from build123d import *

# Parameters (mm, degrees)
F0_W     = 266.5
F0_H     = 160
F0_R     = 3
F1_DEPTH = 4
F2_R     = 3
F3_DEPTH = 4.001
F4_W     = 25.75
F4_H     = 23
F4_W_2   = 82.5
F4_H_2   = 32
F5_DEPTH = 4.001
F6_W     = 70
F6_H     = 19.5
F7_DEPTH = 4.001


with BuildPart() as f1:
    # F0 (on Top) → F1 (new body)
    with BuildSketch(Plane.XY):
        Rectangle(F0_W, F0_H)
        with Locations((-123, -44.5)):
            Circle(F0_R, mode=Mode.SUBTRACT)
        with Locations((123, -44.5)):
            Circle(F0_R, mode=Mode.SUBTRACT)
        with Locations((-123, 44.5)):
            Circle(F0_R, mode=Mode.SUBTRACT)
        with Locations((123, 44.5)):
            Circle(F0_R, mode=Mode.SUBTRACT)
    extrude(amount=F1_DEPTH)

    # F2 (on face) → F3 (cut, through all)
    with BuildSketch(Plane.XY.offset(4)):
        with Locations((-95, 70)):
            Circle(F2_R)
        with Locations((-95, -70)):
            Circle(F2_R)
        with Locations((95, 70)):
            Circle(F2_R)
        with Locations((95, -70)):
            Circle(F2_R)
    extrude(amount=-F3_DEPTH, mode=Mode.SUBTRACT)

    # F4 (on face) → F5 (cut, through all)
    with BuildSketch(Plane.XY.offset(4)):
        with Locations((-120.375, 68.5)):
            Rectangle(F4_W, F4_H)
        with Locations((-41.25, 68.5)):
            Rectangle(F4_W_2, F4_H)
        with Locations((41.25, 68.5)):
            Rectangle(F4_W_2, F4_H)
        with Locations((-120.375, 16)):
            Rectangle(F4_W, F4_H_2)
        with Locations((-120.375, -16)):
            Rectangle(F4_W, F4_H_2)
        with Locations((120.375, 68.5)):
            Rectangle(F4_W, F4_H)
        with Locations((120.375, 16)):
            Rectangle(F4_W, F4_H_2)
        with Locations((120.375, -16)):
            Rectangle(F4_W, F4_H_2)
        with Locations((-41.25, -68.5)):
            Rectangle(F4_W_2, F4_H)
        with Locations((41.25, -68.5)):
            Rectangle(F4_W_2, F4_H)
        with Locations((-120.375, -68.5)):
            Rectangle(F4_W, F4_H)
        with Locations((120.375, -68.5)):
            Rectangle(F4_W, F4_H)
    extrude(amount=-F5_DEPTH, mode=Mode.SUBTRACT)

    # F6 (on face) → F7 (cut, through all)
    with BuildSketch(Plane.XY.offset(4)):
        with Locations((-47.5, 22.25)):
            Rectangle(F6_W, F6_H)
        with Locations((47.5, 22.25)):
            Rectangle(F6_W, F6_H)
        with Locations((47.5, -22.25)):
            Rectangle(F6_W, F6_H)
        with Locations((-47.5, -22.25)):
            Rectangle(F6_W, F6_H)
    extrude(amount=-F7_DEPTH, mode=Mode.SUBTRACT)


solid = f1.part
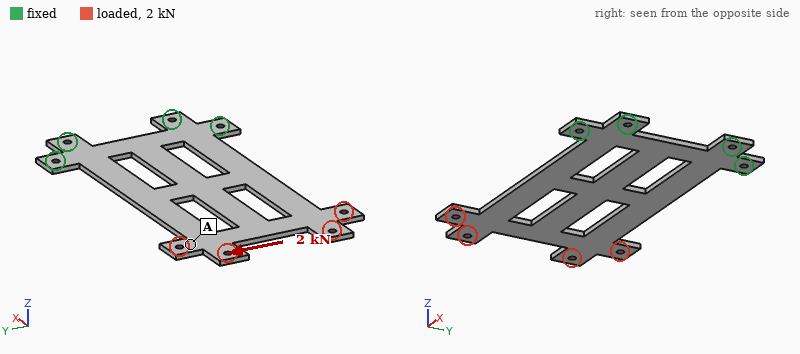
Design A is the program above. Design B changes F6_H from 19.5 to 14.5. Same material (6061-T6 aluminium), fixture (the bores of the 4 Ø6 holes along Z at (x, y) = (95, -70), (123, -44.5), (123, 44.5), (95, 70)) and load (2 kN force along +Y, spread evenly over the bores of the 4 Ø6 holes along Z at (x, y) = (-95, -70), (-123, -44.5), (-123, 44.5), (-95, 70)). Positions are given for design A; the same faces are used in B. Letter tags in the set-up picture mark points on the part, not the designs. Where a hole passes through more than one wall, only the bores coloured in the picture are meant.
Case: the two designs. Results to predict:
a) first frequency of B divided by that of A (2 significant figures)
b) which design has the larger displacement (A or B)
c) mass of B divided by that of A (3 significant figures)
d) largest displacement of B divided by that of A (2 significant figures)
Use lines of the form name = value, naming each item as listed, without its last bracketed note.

first frequency of B divided by that of A = 1.0
which design has the larger displacement = A
mass of B divided by that of A = 1.06
largest displacement of B divided by that of A = 0.85
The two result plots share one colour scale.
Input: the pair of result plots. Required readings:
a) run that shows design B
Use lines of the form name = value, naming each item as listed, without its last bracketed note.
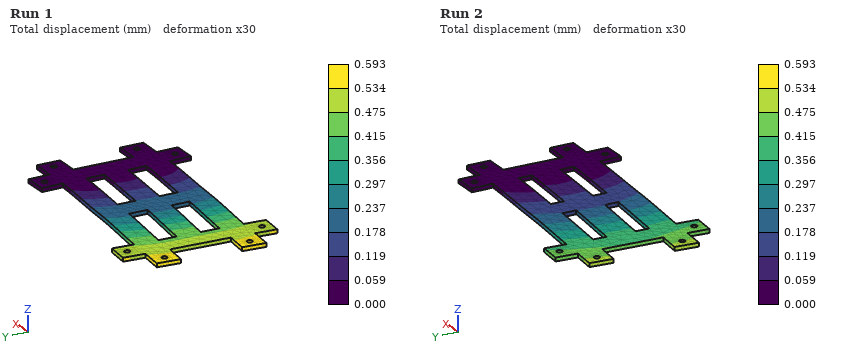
run that shows design B = Run 2
